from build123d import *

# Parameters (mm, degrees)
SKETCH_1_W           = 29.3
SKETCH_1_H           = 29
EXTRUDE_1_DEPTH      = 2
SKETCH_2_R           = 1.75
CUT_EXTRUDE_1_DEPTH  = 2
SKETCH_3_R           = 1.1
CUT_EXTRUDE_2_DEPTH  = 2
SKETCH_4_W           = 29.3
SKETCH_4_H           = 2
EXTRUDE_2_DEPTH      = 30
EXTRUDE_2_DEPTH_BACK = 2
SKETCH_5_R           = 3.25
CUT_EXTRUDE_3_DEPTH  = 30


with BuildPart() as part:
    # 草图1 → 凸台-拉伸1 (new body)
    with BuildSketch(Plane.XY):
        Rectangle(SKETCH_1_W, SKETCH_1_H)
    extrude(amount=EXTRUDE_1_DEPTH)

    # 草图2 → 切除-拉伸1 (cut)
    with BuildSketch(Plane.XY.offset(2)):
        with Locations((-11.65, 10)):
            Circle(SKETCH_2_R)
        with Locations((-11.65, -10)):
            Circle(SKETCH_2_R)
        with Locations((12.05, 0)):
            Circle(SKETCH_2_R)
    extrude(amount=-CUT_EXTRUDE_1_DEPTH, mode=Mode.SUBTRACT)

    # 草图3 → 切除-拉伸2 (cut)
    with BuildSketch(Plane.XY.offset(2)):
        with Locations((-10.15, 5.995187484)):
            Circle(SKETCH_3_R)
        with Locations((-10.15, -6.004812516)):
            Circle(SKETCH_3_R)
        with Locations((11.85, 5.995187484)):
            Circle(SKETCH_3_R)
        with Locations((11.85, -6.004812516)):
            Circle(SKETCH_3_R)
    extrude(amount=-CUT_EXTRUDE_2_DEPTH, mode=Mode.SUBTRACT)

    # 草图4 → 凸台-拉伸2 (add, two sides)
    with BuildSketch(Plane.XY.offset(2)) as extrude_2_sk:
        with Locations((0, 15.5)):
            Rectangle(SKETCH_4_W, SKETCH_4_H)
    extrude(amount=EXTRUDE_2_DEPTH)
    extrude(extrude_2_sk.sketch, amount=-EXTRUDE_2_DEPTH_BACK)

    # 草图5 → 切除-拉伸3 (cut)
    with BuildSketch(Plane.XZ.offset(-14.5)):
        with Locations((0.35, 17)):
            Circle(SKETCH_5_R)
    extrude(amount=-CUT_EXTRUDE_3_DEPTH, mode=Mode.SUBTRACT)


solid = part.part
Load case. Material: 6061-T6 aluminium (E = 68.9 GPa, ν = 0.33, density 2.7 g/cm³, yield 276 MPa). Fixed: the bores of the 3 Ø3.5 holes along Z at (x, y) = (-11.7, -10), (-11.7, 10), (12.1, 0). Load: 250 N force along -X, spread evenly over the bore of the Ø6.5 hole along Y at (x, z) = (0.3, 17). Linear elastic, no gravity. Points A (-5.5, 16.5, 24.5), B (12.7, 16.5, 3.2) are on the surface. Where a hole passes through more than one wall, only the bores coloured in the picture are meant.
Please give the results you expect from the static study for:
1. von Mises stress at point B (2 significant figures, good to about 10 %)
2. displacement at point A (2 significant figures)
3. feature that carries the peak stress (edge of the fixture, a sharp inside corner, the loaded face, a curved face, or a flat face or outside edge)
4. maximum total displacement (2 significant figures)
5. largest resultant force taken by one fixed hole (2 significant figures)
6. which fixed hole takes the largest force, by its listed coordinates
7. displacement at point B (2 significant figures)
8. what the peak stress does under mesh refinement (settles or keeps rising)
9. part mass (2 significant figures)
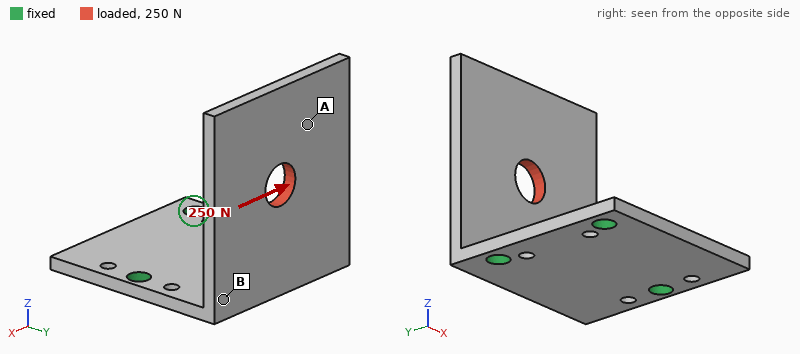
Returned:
45 MPa
0.21 mm
edge of the fixture
0.37 mm
230 N
(-11.7, 10)
0.17 mm
keeps rising
9.2 g
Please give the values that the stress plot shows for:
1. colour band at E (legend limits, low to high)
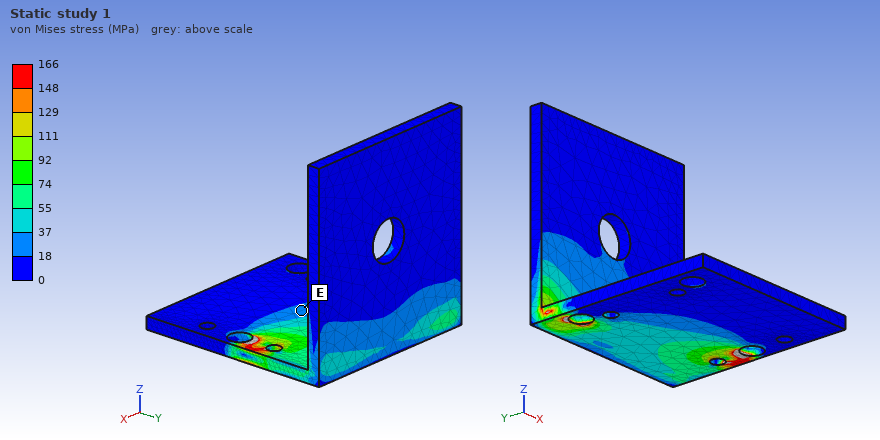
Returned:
18 to 37 MPa
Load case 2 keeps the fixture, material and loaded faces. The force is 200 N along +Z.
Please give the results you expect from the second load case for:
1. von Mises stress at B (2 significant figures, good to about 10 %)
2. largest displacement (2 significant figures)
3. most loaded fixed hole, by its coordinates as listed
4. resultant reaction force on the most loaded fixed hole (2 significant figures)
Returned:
20 MPa
0.26 mm
(-11.7, 10)
150 N
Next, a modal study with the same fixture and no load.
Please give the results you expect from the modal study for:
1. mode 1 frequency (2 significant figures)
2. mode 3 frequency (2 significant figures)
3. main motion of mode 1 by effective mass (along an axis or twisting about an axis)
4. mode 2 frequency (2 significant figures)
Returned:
1200 Hz
4000 Hz
along Y
2700 Hz
